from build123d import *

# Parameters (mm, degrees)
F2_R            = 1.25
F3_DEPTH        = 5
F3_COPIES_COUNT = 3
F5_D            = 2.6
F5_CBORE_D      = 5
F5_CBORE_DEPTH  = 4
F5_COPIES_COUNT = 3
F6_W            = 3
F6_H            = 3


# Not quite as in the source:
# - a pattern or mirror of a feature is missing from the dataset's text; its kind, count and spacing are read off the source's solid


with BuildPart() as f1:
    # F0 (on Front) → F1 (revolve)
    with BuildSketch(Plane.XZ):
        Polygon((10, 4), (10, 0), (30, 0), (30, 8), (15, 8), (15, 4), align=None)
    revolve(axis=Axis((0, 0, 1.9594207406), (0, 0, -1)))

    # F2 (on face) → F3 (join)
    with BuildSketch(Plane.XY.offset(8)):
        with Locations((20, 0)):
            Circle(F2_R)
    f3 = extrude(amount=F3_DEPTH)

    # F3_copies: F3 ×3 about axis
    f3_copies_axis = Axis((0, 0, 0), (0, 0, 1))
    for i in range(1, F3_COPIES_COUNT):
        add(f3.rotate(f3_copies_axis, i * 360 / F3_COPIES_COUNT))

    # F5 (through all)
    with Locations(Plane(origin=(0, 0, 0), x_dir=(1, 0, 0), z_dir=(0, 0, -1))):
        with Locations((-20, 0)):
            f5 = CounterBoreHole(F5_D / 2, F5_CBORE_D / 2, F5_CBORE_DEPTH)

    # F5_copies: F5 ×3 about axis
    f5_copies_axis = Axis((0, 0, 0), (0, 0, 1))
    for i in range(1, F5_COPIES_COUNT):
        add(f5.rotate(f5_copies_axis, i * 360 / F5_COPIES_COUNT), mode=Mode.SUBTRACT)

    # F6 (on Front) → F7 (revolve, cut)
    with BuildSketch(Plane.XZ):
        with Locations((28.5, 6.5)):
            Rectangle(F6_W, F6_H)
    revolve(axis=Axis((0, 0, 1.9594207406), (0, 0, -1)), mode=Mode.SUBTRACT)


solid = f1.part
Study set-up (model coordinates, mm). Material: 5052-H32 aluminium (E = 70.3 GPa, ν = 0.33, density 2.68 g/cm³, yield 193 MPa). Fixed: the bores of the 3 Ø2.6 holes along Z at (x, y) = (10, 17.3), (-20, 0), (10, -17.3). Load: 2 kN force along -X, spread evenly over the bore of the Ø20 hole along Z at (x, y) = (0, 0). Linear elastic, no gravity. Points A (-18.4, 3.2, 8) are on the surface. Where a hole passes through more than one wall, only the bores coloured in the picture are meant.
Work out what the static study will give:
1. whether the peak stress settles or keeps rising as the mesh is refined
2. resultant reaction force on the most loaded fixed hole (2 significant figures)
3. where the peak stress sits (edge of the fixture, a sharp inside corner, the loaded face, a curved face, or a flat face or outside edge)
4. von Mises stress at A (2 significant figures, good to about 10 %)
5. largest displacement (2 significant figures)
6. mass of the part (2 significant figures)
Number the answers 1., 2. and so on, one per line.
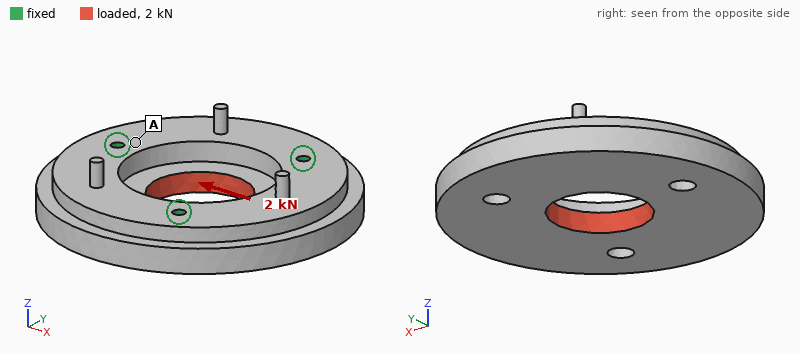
1. keeps rising
2. 700 N
3. edge of the fixture
4. 9.0 MPa
5. 12 µm
6. 45 g
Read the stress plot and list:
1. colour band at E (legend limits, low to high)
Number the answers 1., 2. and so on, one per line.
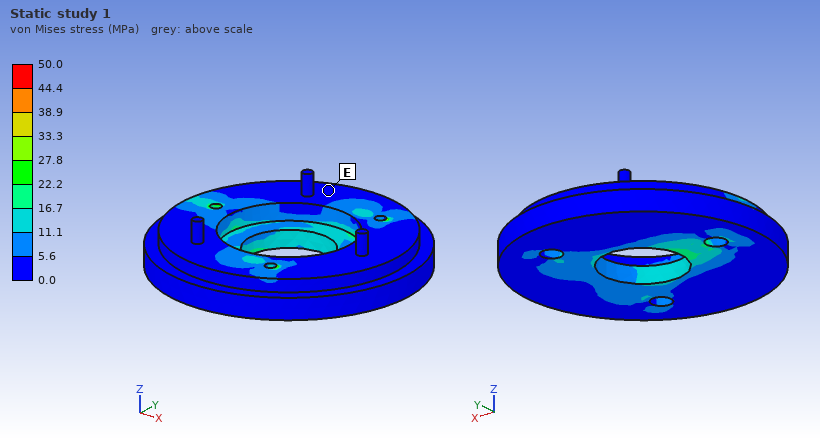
1. 0.0 to 5.6 MPa
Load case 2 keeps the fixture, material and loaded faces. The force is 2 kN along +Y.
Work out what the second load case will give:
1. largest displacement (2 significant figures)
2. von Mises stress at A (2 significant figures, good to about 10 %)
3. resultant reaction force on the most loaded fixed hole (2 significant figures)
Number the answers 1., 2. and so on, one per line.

1. 10 µm
2. 12 MPa
3. 710 N
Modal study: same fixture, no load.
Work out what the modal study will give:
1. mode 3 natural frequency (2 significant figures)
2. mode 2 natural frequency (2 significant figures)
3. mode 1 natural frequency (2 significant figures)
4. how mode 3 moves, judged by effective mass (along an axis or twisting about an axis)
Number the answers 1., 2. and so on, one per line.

1. 13 kHz
2. 8600 Hz
3. 8600 Hz
4. along Z
